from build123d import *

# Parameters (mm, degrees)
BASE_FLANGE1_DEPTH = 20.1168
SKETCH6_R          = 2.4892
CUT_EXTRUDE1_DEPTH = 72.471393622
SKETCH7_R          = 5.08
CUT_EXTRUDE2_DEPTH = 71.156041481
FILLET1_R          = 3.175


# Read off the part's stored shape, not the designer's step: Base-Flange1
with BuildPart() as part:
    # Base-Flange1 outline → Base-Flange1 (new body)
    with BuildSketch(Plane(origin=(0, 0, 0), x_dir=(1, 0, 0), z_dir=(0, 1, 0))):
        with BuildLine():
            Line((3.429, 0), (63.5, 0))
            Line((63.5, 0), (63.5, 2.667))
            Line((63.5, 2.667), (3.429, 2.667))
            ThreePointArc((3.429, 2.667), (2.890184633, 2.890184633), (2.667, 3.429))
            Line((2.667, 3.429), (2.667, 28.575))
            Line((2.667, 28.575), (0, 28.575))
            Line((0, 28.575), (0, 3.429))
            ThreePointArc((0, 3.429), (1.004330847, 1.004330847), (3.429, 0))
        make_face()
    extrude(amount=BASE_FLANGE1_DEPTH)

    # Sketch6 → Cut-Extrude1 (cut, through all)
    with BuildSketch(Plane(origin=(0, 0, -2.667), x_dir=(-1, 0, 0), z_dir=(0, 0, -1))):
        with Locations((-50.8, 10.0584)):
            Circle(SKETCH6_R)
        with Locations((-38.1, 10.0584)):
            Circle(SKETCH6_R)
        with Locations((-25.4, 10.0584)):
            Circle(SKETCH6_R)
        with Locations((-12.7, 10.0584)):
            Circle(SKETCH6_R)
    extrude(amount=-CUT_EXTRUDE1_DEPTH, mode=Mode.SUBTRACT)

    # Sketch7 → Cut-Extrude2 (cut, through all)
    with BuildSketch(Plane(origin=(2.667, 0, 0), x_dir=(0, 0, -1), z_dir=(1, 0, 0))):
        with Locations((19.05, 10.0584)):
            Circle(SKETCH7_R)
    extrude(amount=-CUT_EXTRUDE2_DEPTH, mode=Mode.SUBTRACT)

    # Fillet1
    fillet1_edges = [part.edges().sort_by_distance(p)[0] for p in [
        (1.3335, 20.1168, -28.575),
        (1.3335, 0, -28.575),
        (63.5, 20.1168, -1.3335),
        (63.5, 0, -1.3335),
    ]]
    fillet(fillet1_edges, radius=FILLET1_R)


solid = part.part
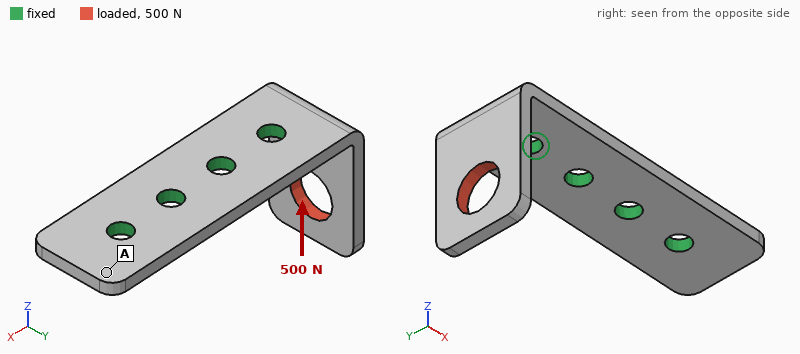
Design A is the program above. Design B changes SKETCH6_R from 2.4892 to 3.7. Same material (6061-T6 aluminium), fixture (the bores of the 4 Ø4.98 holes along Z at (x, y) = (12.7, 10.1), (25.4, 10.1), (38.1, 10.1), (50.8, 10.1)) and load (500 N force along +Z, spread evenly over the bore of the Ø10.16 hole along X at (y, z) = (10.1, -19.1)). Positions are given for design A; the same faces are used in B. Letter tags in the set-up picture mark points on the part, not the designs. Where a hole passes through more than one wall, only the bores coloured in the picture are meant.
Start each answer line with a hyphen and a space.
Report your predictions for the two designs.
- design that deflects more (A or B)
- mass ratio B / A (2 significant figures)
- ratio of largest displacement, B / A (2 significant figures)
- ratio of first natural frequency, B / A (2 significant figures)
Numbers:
- A
- 0.94
- 0.74
- 1.1
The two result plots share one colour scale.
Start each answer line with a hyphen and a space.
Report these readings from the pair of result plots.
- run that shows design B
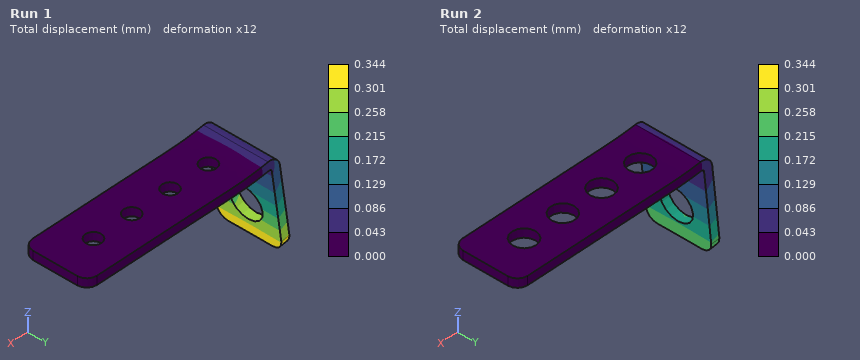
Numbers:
- Run 2
